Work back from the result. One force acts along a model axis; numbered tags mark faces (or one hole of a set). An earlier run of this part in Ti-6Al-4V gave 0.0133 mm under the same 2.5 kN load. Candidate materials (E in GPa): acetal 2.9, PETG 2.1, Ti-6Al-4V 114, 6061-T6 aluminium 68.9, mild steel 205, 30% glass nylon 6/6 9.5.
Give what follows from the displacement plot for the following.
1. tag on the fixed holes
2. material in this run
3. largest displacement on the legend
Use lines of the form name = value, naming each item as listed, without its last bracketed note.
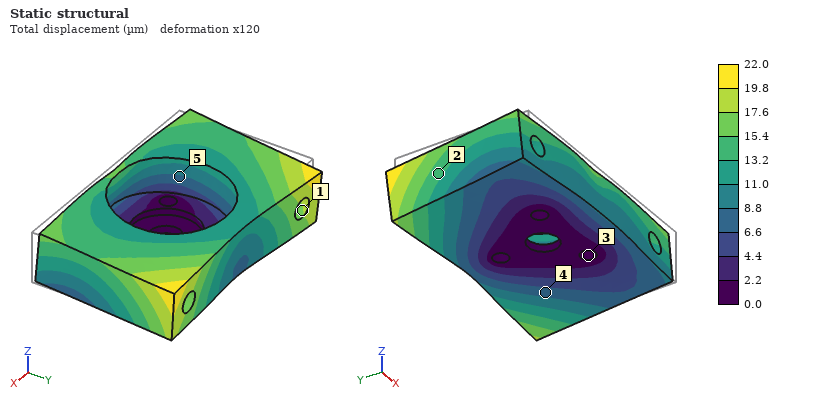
tag on the fixed holes = 3
material in this run = 6061-T6 aluminium
largest displacement on the legend = 22.0 µm
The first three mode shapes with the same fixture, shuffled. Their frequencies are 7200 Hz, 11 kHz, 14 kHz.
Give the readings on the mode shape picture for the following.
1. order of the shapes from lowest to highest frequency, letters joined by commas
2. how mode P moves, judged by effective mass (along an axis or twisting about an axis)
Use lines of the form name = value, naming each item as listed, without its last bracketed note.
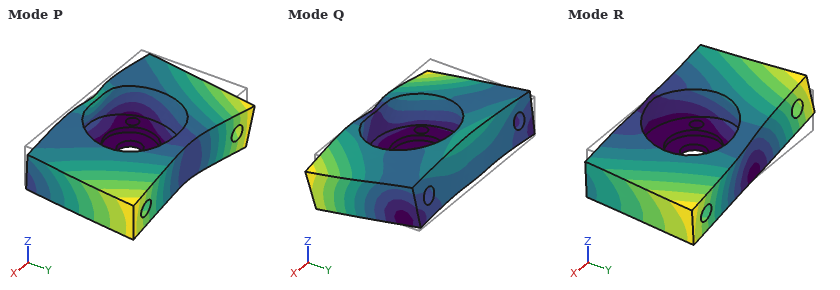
order of the shapes from lowest to highest frequency, letters joined by commas = R, P, Q
how mode P moves, judged by effective mass = along Z
